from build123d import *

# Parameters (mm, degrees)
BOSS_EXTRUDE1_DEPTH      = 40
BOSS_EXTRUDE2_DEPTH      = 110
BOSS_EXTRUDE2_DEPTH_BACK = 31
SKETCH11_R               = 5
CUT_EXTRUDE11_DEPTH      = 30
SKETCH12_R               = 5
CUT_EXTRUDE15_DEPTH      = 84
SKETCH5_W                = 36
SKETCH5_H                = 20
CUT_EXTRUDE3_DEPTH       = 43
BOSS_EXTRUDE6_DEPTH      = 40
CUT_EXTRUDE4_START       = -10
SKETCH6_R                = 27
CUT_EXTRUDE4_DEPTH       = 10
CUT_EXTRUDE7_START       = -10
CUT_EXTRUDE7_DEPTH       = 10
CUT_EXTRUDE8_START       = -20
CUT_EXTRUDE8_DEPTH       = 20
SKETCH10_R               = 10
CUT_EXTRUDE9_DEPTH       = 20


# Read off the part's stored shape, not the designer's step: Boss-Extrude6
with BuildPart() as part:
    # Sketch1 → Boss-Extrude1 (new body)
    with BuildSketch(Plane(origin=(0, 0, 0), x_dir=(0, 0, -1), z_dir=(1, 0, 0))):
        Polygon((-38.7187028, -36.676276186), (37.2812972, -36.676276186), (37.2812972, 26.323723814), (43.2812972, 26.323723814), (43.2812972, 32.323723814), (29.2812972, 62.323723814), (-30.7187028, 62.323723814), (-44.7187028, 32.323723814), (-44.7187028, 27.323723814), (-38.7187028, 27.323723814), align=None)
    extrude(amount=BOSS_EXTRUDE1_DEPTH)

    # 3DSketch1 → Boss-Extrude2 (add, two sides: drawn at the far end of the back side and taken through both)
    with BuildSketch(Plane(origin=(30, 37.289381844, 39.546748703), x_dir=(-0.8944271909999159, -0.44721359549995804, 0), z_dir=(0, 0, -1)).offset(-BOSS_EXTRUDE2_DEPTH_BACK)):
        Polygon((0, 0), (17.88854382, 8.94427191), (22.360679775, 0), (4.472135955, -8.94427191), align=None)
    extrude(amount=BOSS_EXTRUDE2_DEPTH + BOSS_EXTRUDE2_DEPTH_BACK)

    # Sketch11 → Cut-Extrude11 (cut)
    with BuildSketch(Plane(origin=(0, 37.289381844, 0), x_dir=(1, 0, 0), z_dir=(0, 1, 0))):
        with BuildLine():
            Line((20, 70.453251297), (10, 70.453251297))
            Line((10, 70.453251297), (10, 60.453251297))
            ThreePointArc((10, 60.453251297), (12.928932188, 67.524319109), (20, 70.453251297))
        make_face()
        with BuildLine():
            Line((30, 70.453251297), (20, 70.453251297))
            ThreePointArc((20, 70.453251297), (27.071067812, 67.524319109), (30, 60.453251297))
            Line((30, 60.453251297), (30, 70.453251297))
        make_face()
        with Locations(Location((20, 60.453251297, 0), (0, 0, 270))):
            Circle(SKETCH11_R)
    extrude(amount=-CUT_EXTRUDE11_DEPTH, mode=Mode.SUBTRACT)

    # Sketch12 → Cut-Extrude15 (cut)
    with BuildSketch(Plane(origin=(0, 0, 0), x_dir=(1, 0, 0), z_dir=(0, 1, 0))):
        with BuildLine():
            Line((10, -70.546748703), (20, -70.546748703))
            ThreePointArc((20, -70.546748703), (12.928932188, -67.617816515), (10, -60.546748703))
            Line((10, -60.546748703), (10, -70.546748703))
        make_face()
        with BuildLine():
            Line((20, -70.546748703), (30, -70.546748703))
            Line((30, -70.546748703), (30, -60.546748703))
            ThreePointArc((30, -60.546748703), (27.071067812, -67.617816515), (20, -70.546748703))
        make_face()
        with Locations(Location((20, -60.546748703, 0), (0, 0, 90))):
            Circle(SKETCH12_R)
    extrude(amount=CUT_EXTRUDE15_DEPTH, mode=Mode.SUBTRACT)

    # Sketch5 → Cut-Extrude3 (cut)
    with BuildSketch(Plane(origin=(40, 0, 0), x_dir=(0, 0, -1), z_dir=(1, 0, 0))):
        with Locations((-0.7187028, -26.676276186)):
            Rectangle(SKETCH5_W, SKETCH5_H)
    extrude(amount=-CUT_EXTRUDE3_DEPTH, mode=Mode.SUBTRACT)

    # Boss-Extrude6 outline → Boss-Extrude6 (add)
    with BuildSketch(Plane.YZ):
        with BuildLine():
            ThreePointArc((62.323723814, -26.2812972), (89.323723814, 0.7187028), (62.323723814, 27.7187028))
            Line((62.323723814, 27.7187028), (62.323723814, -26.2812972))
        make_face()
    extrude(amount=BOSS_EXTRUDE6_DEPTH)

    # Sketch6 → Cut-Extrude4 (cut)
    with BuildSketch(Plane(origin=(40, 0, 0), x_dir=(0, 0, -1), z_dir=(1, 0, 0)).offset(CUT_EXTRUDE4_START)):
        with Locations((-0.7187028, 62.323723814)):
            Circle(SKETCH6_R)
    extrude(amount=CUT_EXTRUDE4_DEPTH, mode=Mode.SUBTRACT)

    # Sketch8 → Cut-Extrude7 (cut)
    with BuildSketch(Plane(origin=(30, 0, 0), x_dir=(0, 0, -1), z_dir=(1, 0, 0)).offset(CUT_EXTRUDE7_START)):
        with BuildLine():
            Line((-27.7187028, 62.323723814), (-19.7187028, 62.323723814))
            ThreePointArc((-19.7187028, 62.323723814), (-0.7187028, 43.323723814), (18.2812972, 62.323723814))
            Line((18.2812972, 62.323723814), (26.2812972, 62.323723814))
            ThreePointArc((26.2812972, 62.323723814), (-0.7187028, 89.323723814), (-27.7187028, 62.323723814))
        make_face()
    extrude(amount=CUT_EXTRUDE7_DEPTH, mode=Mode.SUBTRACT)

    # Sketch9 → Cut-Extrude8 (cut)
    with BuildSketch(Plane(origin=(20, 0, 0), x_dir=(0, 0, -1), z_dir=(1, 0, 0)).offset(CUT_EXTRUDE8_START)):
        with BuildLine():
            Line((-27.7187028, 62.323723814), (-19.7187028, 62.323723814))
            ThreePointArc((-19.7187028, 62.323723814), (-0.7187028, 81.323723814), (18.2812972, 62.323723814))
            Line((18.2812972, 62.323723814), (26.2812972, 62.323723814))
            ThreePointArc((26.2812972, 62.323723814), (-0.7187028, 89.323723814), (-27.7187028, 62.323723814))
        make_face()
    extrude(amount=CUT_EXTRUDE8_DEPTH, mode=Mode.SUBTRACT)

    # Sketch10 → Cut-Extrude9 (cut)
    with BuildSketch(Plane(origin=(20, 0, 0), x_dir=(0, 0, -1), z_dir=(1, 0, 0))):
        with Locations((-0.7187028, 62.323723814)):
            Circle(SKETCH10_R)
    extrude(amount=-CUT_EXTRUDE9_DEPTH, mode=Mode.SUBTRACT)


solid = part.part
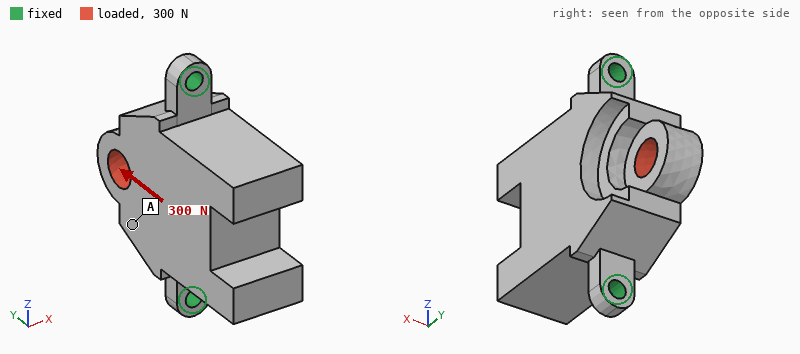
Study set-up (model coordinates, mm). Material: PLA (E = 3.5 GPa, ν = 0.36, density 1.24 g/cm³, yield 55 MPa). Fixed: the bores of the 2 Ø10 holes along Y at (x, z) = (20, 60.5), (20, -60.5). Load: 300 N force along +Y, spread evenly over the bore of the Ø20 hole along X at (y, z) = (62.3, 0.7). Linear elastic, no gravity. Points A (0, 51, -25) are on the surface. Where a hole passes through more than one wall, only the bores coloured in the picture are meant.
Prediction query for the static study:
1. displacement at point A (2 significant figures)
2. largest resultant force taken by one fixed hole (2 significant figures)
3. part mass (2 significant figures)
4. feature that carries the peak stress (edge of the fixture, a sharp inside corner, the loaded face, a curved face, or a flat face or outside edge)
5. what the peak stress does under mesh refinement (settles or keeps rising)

0.12 mm
150 N
330 g
edge of the fixture
keeps rising
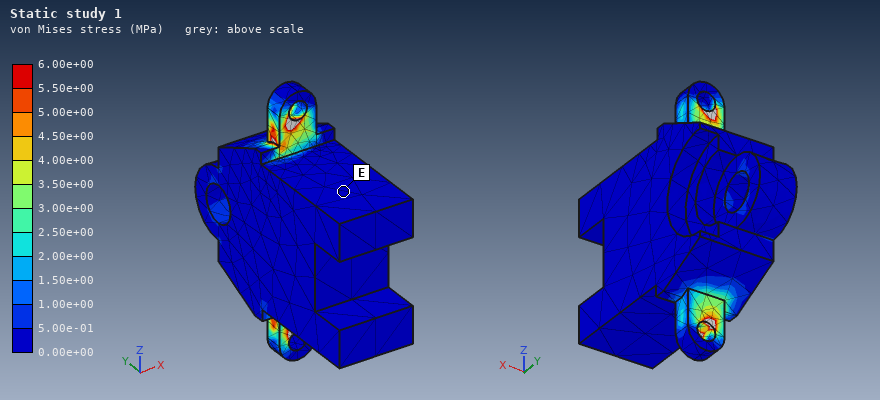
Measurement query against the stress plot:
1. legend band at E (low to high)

0.00e+00 to 5.00e-01 MPa
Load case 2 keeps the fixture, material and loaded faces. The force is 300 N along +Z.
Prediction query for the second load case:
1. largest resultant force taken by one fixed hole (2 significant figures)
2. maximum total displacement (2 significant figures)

180 N
31 µm
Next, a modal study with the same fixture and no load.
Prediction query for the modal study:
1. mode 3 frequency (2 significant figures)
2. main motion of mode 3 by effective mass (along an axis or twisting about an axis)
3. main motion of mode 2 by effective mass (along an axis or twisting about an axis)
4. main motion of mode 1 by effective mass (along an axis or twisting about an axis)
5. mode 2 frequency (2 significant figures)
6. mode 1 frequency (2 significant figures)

1100 Hz
along Z
along Y
along X
900 Hz
240 Hz
